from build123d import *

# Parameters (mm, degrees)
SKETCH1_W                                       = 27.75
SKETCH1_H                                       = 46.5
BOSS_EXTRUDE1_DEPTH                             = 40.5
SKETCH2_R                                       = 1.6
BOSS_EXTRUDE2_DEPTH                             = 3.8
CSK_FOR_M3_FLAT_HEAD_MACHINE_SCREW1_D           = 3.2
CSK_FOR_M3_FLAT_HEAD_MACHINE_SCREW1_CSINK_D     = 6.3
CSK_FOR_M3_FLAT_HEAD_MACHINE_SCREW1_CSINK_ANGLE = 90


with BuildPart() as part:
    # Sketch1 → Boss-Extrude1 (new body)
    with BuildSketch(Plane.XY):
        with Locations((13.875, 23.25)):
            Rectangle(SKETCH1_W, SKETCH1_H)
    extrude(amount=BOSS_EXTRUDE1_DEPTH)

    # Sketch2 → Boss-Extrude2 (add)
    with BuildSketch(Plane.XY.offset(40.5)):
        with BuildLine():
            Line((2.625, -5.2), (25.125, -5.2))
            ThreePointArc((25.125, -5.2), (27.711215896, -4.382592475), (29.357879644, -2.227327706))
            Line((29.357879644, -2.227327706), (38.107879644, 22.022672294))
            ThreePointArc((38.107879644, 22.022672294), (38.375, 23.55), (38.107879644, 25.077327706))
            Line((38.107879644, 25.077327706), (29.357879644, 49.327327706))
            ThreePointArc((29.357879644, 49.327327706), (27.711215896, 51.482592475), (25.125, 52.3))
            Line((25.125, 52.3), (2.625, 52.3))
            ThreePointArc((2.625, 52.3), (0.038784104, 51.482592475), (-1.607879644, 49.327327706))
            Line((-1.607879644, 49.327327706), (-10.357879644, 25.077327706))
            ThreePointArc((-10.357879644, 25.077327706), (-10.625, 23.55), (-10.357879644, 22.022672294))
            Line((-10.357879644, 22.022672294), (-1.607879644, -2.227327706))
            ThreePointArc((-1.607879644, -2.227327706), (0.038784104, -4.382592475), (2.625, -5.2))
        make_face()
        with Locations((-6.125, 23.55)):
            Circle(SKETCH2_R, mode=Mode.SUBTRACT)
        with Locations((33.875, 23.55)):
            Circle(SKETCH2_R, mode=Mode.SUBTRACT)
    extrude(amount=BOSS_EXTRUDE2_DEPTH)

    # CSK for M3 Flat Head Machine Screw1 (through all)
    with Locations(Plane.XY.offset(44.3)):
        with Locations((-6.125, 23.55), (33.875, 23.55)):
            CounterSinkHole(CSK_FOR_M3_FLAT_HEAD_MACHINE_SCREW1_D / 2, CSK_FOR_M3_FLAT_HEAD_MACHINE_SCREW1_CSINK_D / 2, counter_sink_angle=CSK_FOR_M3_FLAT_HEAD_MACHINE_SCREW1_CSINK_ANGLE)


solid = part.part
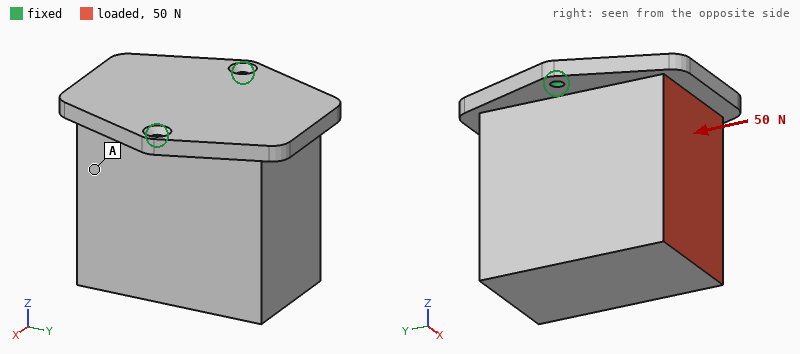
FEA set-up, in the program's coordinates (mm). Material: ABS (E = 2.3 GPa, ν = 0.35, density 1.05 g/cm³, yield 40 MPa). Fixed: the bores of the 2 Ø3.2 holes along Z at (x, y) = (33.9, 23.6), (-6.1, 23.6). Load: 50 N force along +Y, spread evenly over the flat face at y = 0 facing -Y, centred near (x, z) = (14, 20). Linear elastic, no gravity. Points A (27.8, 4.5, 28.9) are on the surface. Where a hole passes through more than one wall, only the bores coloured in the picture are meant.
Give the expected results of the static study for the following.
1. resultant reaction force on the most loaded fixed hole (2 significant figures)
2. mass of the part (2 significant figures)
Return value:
25 N
64 g
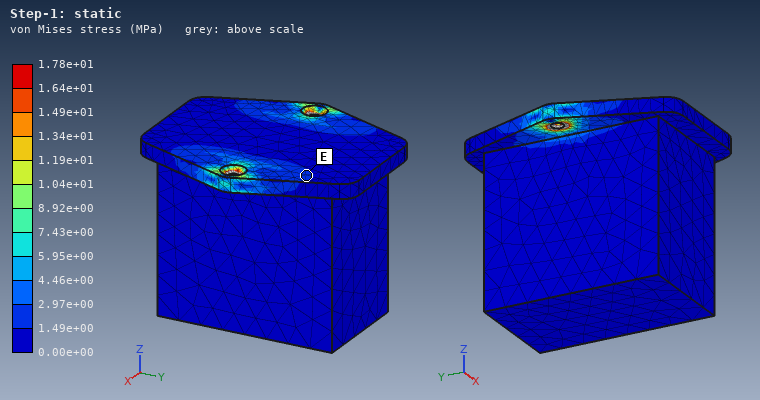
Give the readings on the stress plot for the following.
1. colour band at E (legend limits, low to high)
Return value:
1.49e+00 to 2.97e+00 MPa
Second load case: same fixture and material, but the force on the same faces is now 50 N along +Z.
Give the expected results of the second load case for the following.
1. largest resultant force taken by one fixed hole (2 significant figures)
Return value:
25 N
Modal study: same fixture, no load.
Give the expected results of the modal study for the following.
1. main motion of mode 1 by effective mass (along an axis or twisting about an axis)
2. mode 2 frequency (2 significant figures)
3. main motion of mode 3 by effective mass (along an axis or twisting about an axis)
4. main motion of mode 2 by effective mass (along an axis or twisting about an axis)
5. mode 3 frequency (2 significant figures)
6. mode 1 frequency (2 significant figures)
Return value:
along Y
790 Hz
along Z
along X
1100 Hz
180 Hz
